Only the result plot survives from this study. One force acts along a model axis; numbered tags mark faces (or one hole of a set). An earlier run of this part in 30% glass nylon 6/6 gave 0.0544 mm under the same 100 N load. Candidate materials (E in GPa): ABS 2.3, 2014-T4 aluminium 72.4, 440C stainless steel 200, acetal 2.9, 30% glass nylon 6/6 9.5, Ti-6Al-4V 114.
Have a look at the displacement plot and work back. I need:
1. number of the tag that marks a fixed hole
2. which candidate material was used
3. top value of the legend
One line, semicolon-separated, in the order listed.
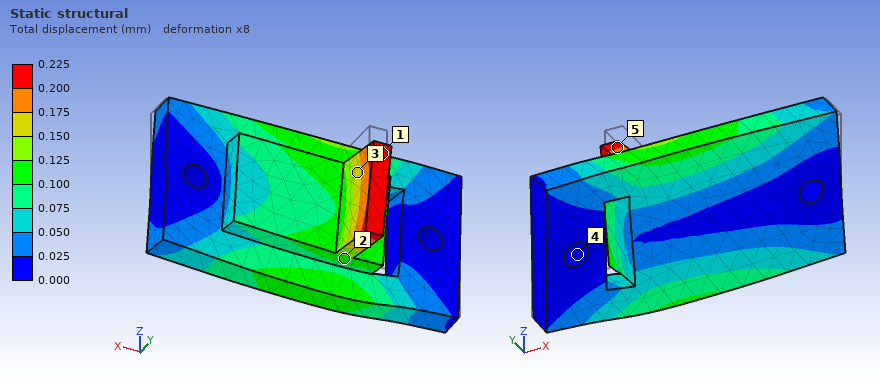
4; ABS; 0.225 mm
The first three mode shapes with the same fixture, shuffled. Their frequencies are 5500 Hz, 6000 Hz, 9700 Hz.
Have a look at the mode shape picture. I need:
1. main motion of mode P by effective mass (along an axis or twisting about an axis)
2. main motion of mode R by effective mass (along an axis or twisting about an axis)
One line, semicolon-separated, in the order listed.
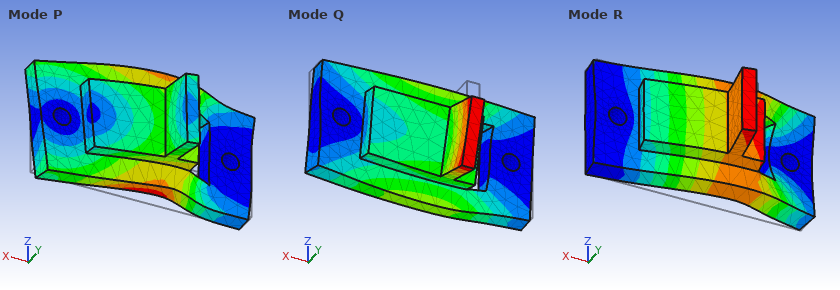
along Z; along Y
